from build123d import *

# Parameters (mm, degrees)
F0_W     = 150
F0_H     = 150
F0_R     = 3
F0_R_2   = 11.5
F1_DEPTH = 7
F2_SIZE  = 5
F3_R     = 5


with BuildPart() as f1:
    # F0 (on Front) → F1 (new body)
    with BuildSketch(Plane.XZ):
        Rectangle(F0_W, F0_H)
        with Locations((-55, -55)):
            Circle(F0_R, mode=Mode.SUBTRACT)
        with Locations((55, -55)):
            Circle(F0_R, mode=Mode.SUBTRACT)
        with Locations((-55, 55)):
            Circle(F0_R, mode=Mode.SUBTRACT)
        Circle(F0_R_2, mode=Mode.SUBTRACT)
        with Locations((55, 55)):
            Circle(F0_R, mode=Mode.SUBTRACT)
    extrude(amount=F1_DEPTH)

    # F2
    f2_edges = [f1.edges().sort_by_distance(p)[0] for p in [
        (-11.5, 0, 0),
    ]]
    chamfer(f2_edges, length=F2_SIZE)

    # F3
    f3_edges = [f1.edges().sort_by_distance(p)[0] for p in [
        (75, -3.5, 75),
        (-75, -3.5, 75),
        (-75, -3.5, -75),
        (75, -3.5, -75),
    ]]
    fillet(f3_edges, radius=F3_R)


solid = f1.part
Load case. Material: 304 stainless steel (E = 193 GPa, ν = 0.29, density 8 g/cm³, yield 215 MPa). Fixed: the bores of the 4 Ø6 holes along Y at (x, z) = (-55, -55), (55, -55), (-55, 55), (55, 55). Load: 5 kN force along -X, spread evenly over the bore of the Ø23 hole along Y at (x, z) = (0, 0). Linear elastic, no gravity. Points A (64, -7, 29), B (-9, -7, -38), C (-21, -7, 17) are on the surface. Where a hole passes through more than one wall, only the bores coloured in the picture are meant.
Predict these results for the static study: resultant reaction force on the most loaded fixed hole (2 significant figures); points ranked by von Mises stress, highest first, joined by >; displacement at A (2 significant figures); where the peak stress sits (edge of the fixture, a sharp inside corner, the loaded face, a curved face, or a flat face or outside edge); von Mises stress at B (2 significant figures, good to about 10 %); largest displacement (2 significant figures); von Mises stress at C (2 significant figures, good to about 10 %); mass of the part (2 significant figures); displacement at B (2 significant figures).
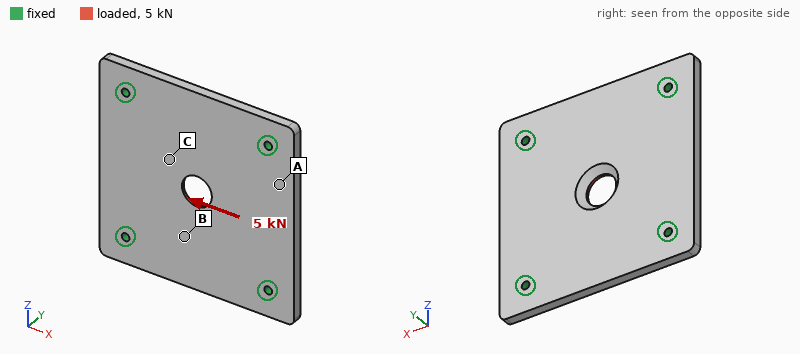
1.4 kN
C > B > A
1.7 µm
the loaded face
6.2 MPa
4.3 µm
10 MPa
1.2 kg
1.5 µm
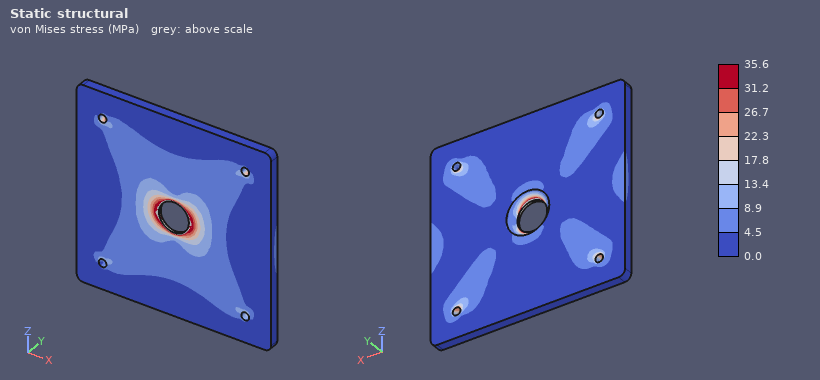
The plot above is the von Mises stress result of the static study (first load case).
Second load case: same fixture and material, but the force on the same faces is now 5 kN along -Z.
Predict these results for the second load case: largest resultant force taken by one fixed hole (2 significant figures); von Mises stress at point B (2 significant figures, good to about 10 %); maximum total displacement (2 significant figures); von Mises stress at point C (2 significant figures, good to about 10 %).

1.4 kN
5.3 MPa
4.3 µm
9.5 MPa
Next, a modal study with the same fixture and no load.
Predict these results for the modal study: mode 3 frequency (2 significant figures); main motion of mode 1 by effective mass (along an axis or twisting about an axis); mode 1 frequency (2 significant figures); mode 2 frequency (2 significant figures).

2900 Hz
along Y
1900 Hz
2900 Hz
